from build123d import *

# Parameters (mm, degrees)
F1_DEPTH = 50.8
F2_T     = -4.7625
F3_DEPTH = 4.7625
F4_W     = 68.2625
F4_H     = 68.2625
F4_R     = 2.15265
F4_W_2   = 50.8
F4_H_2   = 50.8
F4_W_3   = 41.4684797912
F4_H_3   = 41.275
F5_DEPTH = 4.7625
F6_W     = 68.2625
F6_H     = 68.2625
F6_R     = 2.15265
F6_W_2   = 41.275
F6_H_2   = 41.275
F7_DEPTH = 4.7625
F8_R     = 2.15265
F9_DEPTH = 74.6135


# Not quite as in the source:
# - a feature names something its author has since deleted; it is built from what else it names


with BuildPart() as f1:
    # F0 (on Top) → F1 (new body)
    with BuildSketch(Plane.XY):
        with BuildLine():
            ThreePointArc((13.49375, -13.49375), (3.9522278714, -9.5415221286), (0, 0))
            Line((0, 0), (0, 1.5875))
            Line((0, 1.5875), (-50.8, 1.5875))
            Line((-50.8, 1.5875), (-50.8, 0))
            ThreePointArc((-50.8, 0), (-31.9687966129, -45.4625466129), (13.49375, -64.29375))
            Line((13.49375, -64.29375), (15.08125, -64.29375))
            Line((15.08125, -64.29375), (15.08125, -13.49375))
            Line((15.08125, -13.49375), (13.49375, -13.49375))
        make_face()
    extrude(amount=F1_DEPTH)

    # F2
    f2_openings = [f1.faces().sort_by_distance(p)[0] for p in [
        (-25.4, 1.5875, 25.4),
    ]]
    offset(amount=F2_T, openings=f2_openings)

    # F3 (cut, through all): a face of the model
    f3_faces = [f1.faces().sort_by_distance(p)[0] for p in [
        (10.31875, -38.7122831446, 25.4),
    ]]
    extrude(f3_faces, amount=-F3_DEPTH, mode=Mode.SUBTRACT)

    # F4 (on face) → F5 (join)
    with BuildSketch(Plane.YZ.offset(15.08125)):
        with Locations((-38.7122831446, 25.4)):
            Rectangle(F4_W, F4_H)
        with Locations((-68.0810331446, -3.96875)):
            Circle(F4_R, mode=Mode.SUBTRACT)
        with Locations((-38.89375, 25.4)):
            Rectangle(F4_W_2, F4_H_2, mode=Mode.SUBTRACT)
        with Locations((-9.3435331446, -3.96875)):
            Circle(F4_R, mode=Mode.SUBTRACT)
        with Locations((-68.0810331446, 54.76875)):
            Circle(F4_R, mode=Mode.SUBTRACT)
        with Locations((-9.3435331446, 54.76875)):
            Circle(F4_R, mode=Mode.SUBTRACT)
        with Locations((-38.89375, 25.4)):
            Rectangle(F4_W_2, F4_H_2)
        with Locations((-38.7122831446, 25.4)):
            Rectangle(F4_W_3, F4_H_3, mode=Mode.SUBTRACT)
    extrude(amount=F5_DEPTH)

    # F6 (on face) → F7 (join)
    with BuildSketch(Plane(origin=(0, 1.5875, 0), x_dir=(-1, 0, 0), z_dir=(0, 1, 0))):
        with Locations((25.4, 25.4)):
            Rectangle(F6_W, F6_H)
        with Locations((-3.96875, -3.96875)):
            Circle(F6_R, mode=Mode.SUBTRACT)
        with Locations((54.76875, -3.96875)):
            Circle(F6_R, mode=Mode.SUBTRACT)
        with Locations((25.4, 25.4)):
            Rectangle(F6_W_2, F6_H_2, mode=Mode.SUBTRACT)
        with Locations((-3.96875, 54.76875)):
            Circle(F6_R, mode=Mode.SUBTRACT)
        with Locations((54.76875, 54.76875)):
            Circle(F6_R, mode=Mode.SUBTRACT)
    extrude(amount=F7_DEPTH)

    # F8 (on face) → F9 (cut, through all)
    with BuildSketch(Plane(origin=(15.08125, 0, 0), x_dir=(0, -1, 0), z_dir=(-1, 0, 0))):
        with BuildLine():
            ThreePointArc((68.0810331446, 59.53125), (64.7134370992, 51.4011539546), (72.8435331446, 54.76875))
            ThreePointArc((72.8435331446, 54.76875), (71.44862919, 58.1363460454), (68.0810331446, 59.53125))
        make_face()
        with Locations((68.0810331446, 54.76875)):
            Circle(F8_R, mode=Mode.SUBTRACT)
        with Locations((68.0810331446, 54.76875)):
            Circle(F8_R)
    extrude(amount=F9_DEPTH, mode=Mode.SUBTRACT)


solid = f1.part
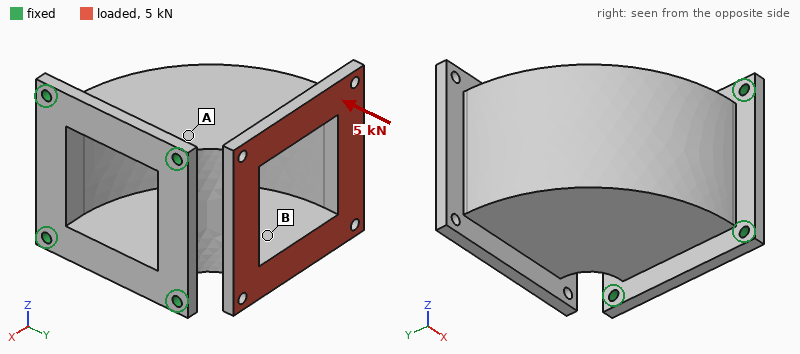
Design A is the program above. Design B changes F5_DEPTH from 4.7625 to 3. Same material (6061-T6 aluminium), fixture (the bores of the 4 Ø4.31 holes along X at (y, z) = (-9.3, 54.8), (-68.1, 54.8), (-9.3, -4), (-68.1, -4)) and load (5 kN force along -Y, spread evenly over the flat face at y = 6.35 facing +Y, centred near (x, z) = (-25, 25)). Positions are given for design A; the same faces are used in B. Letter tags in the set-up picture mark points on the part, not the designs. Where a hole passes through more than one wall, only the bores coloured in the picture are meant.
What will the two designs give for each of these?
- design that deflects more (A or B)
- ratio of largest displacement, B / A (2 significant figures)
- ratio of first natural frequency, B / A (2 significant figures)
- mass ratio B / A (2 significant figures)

B
1.6
0.83
0.94
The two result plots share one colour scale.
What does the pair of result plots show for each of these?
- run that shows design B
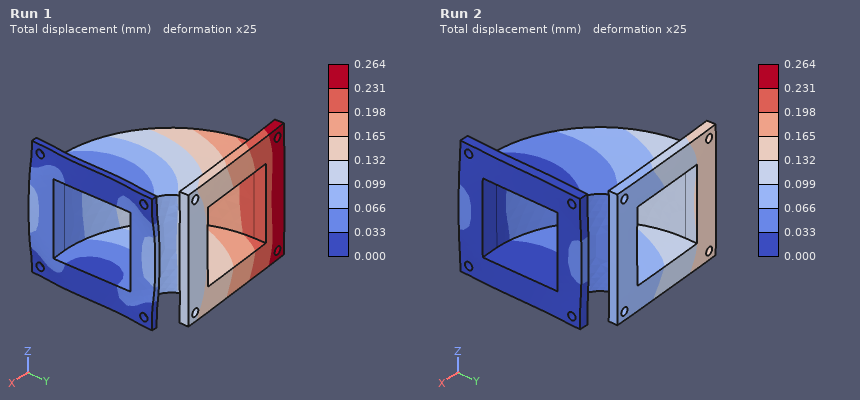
Run 1
